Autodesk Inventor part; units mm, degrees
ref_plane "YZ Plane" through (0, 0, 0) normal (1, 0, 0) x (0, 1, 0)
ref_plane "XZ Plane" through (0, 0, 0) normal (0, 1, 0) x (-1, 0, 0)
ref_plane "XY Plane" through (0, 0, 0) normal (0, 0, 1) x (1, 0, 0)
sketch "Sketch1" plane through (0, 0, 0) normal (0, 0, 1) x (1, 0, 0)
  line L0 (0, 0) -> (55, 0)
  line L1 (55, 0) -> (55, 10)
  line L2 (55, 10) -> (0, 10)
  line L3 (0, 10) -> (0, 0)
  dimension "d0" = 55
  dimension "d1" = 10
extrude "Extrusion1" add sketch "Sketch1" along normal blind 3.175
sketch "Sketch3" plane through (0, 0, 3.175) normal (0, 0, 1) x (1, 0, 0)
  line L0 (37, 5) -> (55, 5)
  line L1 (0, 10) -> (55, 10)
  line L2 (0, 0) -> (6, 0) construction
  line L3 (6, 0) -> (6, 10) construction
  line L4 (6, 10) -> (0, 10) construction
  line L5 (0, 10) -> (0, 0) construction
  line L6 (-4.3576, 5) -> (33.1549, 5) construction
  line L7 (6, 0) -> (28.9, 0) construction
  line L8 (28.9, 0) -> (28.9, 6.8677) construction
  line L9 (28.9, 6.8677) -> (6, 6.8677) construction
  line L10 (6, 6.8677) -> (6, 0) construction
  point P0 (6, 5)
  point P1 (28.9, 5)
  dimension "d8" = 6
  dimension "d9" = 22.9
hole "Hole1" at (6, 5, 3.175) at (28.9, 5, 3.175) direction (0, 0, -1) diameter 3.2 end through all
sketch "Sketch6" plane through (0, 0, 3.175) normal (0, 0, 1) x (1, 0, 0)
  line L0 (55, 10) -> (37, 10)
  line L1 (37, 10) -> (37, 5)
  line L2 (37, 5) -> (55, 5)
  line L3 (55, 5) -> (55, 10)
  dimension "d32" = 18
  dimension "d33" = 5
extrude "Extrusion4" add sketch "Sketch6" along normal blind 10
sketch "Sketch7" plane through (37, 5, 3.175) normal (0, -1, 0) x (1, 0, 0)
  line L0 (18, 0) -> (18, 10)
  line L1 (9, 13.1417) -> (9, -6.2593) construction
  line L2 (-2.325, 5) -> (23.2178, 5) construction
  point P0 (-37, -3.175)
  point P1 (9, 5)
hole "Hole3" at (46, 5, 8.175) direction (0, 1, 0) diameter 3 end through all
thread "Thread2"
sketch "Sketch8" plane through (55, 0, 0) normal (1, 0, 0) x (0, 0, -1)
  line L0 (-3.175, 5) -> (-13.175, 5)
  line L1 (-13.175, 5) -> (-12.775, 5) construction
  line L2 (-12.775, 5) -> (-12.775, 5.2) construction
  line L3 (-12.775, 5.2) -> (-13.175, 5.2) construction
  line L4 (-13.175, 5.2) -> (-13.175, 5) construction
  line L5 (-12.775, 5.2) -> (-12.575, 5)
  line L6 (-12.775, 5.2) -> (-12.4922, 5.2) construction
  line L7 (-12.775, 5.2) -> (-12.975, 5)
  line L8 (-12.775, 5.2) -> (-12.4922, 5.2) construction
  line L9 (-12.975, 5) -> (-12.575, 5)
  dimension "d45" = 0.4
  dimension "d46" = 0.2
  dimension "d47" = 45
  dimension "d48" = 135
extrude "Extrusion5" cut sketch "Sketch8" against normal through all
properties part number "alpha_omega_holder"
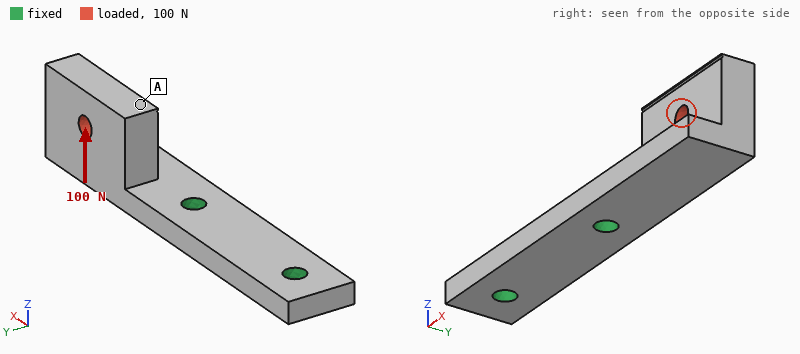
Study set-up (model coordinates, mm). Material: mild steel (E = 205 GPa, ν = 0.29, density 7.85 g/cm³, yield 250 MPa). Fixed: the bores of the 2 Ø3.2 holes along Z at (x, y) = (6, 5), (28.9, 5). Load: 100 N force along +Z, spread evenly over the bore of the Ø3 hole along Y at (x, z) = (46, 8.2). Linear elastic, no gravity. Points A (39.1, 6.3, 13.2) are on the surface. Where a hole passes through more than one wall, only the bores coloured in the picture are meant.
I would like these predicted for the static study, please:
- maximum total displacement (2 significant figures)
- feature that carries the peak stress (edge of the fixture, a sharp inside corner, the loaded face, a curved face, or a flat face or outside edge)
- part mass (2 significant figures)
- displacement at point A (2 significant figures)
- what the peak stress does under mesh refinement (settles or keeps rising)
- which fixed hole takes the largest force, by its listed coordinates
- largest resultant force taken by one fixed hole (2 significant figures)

53 µm
edge of the fixture
20 g
27 µm
keeps rising
(28.9, 5)
100 N
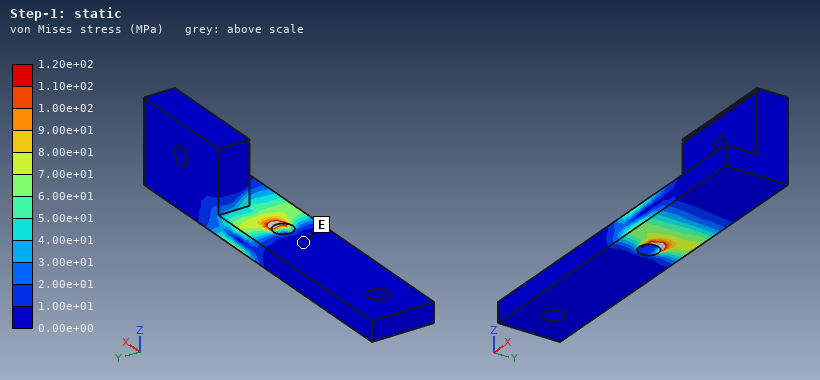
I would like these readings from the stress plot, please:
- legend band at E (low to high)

0.00e+00 to 1.00e+01 MPa
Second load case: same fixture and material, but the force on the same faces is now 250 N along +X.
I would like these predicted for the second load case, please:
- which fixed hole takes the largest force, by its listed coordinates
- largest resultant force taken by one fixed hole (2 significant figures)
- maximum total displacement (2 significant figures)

(28.9, 5)
240 N
71 µm
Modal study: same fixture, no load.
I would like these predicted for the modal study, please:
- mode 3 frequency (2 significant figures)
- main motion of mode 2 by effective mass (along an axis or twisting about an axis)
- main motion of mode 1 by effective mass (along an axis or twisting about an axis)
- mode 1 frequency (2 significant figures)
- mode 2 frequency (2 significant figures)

9700 Hz
along Y
along Z
2500 Hz
5000 Hz
